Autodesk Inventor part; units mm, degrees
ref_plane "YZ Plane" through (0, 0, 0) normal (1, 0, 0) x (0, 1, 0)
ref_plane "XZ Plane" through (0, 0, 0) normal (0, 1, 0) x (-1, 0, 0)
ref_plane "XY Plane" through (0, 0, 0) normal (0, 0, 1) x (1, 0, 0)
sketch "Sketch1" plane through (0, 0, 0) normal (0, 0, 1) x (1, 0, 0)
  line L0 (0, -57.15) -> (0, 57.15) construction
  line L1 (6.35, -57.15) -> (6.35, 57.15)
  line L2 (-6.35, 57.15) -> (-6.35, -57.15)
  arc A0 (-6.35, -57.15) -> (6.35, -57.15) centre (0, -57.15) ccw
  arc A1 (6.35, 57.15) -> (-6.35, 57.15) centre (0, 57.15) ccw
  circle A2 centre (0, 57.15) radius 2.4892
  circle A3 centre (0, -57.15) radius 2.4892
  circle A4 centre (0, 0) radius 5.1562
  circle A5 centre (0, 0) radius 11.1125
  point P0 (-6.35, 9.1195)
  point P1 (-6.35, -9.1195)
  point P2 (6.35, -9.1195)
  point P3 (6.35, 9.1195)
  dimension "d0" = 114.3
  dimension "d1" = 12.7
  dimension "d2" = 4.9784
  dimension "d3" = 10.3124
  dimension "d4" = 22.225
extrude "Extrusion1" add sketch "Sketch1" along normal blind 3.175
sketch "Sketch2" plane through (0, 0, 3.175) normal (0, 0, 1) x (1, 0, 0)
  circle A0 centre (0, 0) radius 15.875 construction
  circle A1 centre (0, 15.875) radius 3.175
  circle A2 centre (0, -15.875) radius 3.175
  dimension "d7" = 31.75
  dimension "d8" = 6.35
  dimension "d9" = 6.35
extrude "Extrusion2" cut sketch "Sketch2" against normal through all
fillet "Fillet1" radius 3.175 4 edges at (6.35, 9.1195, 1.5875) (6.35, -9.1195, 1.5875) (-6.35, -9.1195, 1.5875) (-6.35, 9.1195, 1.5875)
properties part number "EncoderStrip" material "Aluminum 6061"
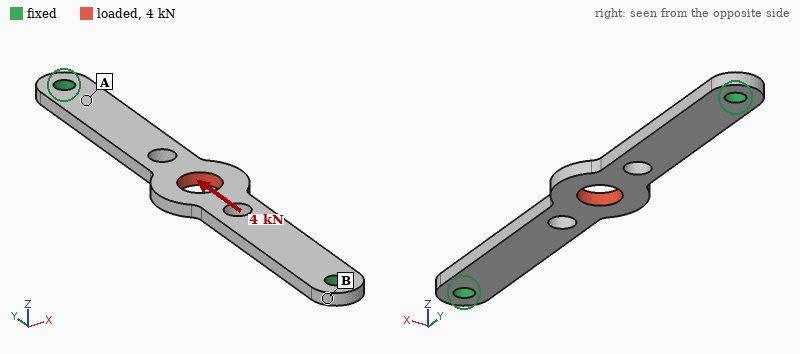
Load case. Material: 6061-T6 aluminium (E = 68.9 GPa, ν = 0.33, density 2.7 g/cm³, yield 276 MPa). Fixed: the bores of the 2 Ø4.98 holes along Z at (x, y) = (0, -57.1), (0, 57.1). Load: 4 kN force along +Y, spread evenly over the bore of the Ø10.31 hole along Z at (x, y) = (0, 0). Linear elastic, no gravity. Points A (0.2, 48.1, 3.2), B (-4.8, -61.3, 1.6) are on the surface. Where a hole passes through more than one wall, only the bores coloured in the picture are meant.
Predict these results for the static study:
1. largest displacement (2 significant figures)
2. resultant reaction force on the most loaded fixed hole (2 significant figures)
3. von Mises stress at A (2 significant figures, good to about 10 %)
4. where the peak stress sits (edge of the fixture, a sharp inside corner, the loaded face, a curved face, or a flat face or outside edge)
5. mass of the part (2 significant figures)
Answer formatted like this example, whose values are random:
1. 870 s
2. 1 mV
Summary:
1. 47 µm
2. 2.0 kN
3. 57 MPa
4. a curved face
5. 13 g
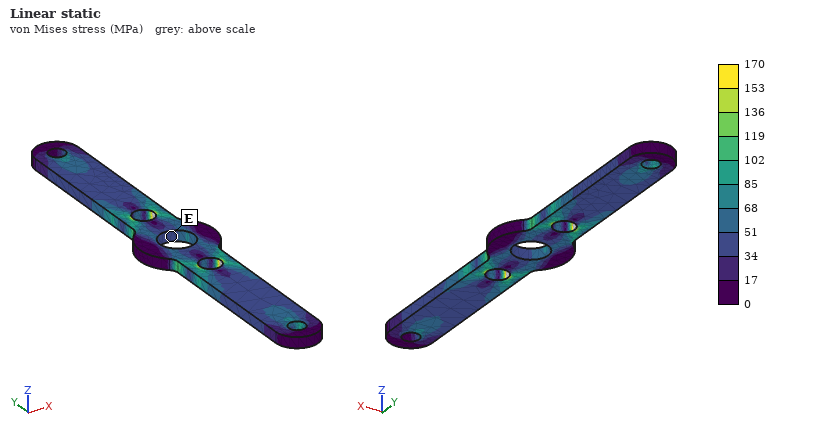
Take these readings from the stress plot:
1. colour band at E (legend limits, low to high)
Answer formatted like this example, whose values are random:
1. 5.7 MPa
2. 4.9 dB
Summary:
1. 34 to 51 MPa
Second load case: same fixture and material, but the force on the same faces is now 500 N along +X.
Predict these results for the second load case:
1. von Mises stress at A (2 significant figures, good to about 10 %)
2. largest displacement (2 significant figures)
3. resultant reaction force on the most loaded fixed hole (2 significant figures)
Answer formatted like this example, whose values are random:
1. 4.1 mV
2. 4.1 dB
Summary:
1. 17 MPa
2. 0.12 mm
3. 250 N
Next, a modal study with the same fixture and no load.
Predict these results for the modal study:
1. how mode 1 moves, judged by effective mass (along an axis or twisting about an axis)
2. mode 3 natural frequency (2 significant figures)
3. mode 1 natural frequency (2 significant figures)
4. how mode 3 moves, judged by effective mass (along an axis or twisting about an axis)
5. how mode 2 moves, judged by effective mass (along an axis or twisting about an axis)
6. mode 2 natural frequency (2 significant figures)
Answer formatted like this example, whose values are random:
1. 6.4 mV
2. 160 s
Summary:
1. along Z
2. 4500 Hz
3. 1300 Hz
4. along X
5. twisting about X
6. 3500 Hz
